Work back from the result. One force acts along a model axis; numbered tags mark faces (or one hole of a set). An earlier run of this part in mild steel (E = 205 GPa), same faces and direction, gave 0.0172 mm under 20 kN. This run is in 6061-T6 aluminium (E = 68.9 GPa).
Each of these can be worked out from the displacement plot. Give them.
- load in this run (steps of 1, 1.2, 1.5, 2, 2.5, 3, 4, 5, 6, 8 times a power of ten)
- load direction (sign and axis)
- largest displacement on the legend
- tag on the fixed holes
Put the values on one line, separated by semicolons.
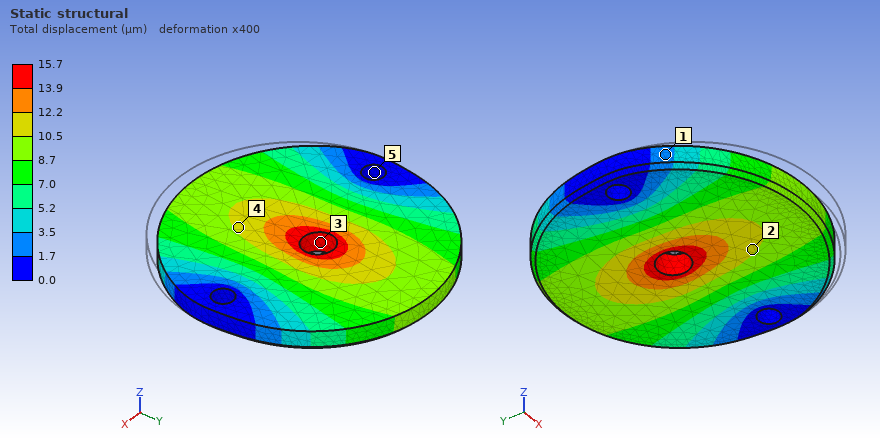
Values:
6 kN; +Y; 15.7 µm; 5
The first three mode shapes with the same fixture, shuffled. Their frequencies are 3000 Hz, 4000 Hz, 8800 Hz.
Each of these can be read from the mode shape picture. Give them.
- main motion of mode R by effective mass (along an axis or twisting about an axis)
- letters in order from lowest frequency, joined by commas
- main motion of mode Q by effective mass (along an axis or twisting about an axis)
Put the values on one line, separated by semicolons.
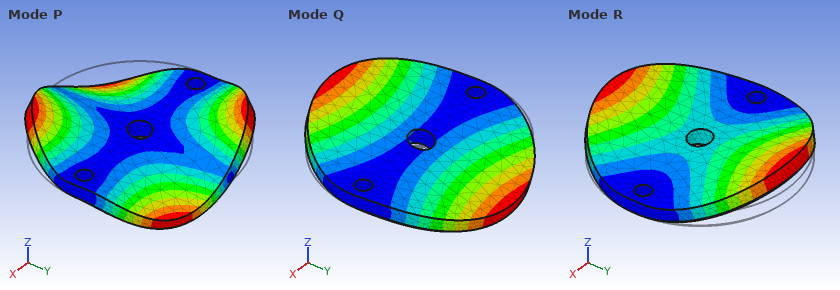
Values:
along Z; Q, R, P; twisting about X
